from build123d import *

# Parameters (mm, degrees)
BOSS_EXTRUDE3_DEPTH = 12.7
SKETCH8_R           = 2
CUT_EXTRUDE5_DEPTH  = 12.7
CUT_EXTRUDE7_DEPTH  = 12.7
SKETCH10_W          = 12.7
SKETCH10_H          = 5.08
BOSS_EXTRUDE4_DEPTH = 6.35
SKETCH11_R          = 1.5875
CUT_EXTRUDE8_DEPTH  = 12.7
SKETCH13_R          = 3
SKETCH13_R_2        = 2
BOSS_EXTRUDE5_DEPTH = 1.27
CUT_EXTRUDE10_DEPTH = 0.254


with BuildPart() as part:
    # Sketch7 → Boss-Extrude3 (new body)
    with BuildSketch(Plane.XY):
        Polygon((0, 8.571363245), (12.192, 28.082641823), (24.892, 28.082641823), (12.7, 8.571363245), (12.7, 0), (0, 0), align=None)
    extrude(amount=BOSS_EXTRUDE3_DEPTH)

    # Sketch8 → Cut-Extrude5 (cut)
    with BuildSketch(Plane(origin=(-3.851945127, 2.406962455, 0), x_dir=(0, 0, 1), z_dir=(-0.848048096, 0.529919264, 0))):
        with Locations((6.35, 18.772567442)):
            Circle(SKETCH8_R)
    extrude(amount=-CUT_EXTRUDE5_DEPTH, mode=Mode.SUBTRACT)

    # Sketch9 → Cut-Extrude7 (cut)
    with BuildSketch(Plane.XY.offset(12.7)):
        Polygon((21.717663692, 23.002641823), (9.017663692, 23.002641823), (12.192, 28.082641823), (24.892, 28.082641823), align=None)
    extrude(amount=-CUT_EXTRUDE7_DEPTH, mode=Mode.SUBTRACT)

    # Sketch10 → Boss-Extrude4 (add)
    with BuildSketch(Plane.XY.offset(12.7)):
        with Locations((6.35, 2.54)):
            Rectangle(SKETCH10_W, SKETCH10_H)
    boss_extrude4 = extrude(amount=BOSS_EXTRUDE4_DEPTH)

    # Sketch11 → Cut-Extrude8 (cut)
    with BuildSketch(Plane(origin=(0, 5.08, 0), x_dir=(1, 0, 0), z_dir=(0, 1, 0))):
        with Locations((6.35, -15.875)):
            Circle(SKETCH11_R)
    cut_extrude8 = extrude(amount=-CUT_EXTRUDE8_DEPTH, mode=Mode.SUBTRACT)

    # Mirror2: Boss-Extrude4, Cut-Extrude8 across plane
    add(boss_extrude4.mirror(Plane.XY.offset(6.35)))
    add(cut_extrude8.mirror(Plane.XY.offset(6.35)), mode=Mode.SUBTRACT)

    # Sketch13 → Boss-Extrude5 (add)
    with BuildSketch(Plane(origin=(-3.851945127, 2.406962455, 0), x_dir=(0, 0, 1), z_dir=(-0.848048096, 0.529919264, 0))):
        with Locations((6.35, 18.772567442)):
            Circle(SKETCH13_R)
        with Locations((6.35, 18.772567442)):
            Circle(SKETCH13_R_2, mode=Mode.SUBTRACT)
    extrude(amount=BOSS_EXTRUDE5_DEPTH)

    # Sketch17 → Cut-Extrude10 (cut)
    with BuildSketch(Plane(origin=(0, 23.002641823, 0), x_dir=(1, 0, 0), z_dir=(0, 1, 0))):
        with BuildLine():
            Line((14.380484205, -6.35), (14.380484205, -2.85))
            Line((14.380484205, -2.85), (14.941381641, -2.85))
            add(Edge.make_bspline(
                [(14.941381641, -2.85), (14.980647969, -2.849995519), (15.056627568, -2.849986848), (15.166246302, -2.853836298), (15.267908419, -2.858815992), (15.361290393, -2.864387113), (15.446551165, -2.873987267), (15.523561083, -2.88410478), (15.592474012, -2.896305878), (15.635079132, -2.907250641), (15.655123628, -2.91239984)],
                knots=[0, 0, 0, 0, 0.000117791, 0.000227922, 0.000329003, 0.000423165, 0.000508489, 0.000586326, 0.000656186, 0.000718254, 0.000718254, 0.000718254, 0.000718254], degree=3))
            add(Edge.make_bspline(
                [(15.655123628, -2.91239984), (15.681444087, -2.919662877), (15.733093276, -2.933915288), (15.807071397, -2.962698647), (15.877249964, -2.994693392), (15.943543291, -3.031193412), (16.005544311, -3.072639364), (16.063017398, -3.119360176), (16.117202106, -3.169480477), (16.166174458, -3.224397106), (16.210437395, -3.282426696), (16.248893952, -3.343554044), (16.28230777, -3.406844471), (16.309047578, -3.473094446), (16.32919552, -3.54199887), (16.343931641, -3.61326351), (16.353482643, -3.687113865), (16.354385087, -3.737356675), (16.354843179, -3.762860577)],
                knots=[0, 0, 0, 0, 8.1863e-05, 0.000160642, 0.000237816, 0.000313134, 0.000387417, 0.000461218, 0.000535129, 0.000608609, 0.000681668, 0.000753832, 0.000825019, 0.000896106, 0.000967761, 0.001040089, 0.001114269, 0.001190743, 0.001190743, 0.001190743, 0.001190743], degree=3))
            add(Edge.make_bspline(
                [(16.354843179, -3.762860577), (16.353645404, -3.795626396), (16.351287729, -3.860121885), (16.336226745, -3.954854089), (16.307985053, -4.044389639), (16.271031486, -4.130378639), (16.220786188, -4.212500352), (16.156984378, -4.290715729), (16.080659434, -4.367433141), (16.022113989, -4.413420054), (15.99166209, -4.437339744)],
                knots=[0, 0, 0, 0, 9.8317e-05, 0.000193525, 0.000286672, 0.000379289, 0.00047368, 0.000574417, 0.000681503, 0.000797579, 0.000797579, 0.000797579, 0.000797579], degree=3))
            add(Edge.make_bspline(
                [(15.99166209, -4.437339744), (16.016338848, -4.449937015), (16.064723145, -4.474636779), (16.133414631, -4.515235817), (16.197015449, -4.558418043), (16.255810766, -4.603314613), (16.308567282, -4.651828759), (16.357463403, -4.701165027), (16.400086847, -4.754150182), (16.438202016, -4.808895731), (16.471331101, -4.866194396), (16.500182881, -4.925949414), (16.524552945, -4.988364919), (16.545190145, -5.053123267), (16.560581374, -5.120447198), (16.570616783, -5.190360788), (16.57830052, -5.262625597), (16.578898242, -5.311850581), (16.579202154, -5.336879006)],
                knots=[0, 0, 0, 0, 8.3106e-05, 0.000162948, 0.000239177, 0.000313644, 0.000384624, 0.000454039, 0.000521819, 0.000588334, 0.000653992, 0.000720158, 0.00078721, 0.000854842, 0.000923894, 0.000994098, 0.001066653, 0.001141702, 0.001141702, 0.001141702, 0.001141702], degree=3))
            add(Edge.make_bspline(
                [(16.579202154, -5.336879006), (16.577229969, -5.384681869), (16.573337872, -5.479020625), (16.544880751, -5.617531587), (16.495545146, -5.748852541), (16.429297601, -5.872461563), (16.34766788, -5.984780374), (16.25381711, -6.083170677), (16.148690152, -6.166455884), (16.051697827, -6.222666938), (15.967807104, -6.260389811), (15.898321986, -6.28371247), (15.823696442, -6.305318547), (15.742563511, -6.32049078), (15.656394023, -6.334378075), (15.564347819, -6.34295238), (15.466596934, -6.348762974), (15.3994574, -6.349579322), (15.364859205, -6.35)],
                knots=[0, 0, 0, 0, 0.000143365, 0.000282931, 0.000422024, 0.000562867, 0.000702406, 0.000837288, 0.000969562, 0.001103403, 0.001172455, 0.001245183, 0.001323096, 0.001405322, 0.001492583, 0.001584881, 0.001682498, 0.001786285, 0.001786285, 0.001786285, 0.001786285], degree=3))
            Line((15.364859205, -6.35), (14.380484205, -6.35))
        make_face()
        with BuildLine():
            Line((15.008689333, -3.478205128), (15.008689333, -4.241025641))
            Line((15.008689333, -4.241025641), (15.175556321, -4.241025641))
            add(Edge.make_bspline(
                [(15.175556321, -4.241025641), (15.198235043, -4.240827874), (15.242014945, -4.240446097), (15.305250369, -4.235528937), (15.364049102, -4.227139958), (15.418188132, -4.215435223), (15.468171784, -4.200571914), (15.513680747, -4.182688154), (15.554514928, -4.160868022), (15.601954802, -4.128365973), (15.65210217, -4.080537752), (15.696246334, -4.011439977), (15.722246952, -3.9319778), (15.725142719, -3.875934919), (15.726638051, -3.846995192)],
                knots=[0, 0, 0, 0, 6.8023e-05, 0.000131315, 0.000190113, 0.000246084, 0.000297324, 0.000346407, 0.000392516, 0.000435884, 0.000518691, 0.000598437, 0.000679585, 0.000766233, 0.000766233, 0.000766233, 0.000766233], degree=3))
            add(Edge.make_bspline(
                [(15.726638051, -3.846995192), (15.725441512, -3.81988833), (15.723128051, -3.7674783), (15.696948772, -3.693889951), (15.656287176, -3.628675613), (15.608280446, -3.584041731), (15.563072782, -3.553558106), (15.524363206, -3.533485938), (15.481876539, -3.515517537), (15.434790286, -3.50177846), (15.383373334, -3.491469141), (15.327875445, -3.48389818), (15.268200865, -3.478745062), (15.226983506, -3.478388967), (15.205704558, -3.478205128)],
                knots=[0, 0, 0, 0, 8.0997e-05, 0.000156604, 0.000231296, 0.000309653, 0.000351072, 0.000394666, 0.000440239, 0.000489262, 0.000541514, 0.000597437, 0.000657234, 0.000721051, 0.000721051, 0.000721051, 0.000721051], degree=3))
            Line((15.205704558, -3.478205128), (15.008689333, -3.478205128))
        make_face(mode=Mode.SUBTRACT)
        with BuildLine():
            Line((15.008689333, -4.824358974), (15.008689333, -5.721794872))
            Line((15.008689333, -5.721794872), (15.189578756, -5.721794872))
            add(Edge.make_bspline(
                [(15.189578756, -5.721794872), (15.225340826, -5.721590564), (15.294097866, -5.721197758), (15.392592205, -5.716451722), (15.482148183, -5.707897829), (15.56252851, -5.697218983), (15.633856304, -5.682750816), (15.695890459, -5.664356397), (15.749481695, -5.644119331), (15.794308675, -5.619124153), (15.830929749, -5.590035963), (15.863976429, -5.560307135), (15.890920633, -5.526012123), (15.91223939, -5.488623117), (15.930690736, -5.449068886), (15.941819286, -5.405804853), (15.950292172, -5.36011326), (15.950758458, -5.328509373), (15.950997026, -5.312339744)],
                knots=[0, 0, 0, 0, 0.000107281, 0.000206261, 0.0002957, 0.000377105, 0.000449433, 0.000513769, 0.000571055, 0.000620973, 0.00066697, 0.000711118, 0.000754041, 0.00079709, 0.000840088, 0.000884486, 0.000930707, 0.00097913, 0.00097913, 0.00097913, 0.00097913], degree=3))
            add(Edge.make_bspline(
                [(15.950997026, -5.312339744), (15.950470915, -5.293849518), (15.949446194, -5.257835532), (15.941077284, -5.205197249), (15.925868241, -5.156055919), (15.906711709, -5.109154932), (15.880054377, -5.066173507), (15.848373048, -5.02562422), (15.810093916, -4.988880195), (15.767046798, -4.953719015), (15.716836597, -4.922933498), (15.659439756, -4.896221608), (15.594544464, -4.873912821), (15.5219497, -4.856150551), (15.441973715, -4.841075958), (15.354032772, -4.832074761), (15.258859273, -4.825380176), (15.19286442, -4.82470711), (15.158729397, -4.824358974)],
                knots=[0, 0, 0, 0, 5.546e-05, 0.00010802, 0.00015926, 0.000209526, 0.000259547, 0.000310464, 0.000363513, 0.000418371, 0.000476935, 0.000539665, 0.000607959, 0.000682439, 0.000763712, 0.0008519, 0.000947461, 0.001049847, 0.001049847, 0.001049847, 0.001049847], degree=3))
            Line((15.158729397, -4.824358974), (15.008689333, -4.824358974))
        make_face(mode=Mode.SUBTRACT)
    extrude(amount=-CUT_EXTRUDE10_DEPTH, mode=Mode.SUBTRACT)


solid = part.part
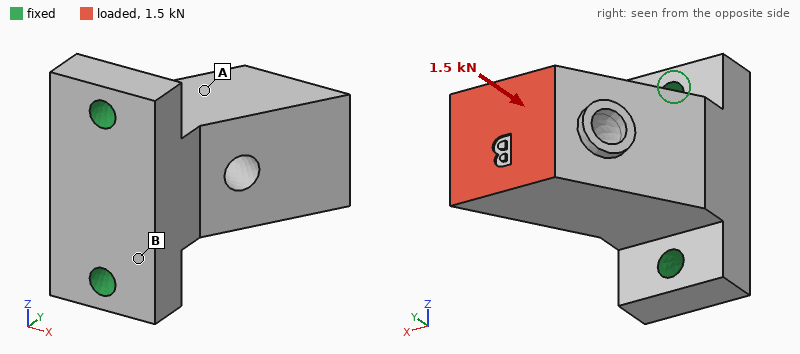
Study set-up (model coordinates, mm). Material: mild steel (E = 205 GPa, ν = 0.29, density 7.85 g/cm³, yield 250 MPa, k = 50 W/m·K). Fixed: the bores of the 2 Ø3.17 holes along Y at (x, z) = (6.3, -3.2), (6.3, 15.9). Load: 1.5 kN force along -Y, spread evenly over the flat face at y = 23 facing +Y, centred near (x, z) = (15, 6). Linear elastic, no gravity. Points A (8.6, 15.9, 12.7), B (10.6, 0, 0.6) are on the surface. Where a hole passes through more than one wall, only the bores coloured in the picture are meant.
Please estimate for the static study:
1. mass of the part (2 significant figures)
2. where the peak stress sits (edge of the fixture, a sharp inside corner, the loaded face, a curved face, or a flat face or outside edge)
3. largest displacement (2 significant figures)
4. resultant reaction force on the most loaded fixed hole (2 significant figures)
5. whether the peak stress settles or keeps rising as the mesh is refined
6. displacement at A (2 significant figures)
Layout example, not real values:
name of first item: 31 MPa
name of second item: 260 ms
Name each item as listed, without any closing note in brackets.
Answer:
mass of the part: 34 g
where the peak stress sits: edge of the fixture
largest displacement: 35 µm
resultant reaction force on the most loaded fixed hole: 790 N
whether the peak stress settles or keeps rising as the mesh is refined: keeps rising
displacement at A: 14 µm
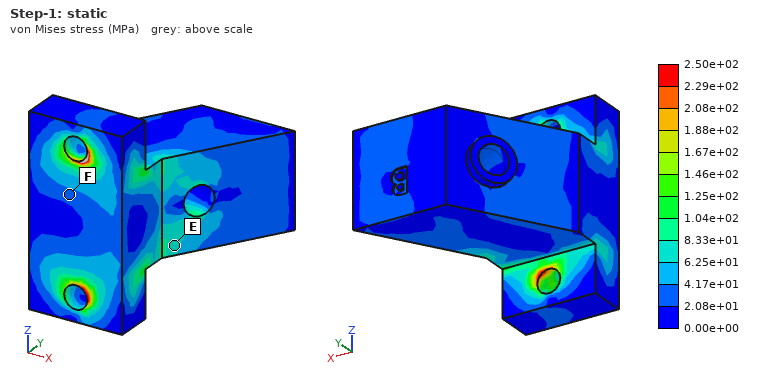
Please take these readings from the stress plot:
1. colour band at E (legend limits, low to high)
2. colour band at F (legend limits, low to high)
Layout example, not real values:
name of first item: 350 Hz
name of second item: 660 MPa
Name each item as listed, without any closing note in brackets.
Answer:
colour band at E: 6.25e+01 to 8.33e+01 MPa
colour band at F: 2.08e+01 to 4.17e+01 MPa
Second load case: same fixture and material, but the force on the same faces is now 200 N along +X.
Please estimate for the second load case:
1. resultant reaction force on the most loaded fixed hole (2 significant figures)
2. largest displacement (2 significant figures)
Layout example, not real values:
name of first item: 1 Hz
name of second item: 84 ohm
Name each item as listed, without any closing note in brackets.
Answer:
resultant reaction force on the most loaded fixed hole: 100 N
largest displacement: 9.5 µm
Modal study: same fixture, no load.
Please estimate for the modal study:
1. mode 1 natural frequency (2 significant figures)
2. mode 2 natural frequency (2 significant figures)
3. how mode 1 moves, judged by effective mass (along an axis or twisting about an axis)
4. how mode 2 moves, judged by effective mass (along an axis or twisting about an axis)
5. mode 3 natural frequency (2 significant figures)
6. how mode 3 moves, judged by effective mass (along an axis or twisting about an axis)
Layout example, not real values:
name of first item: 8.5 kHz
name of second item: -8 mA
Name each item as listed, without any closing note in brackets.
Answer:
mode 1 natural frequency: 8500 Hz
mode 2 natural frequency: 15 kHz
how mode 1 moves, judged by effective mass: along X
how mode 2 moves, judged by effective mass: along Z
mode 3 natural frequency: 29 kHz
how mode 3 moves, judged by effective mass: along Y
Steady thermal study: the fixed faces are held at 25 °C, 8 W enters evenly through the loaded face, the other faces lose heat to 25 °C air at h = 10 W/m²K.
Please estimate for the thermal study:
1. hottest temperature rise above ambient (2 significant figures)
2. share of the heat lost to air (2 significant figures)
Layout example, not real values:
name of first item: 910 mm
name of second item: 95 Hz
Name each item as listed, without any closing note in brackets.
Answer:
hottest temperature rise above ambient: 36 K
share of the heat lost to air: 3.1 %
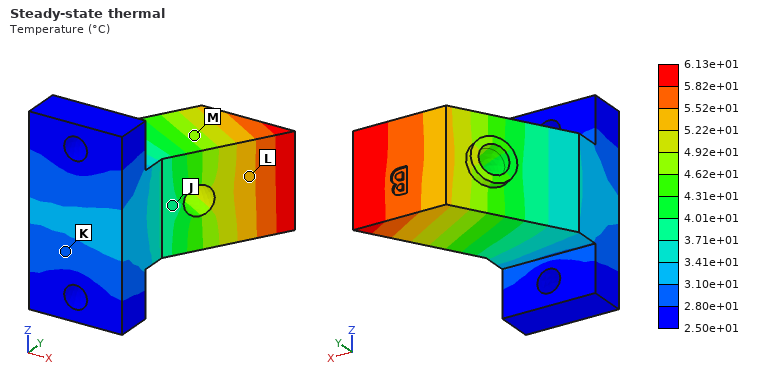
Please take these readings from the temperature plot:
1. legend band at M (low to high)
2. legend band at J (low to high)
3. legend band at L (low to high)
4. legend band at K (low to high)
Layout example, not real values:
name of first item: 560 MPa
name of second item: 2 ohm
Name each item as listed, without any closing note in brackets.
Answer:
legend band at M: 4.62e+01 to 4.92e+01 °C
legend band at J: 3.71e+01 to 4.01e+01 °C
legend band at L: 5.22e+01 to 5.52e+01 °C
legend band at K: 2.80e+01 to 3.10e+01 °C
